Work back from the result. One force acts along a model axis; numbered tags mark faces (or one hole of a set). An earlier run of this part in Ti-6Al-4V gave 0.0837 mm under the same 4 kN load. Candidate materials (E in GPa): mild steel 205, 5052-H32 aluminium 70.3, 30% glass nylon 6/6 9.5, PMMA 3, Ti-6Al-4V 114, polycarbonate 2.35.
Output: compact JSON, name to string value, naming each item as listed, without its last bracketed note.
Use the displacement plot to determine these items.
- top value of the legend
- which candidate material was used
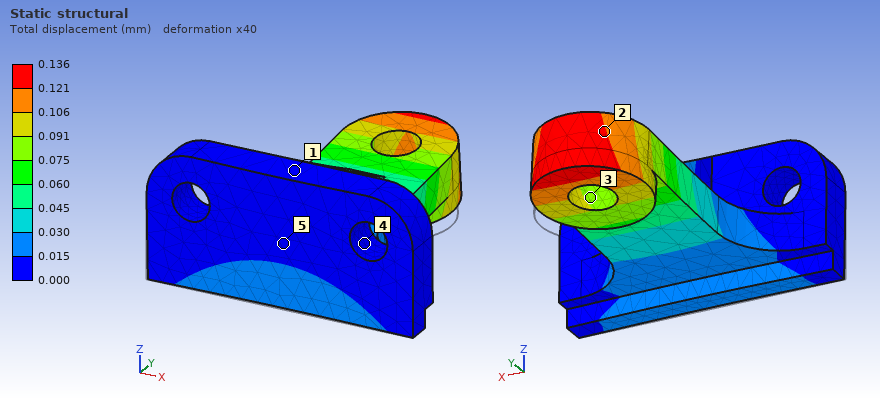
{"top value of the legend": "0.136 mm", "which candidate material was used": "5052-H32 aluminium"}
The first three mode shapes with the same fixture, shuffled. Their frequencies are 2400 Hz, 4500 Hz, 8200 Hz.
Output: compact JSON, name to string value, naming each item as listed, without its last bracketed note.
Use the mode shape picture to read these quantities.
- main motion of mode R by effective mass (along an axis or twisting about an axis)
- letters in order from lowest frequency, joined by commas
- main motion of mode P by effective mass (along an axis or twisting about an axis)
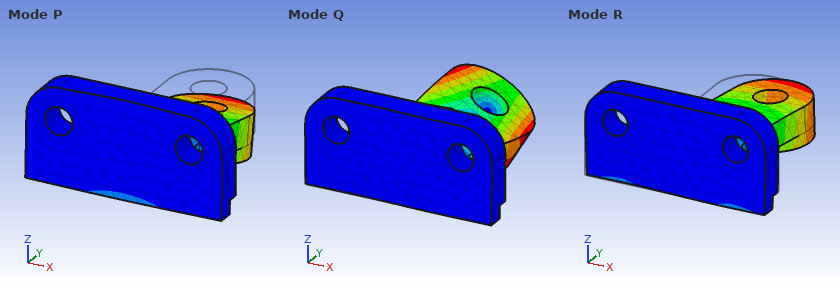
{"main motion of mode R by effective mass": "along X", "letters in order from lowest frequency, joined by commas": "P, R, Q", "main motion of mode P by effective mass": "along Z"}
